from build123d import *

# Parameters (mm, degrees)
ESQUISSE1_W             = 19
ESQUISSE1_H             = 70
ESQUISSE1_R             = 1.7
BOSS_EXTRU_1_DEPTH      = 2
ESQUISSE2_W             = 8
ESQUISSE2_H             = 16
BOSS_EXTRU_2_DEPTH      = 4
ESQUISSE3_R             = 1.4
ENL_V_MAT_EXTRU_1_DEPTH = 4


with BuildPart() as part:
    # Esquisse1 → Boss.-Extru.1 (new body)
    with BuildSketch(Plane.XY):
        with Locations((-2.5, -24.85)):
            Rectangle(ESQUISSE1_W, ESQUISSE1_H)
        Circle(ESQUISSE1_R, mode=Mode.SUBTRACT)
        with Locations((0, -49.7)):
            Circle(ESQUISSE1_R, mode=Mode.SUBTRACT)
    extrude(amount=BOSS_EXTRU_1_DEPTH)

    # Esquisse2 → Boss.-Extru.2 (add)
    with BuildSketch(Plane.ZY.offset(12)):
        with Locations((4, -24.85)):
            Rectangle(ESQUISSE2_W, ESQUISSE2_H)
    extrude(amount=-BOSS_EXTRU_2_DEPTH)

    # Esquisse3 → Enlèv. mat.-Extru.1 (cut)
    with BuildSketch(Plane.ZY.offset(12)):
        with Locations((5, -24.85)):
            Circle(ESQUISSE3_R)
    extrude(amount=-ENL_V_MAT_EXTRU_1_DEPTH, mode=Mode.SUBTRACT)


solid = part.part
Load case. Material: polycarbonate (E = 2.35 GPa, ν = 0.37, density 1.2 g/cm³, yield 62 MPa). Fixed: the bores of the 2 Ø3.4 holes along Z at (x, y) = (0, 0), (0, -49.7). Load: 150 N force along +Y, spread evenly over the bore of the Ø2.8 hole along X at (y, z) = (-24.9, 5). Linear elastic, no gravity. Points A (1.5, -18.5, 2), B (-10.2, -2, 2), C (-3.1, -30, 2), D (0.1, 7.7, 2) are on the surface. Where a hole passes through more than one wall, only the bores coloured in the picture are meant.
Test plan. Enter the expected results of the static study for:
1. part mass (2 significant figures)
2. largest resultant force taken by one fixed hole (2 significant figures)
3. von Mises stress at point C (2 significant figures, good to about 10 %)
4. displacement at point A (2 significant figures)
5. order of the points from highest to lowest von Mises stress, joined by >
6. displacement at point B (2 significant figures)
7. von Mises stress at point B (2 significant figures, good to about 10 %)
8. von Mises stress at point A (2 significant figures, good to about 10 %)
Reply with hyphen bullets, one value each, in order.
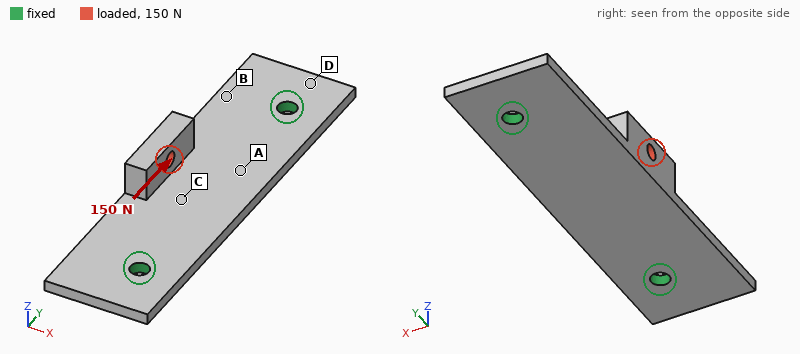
- 3.6 g
- 82 N
- 10 MPa
- 0.090 mm
- C > A > B > D
- 0.12 mm
- 3.6 MPa
- 6.9 MPa
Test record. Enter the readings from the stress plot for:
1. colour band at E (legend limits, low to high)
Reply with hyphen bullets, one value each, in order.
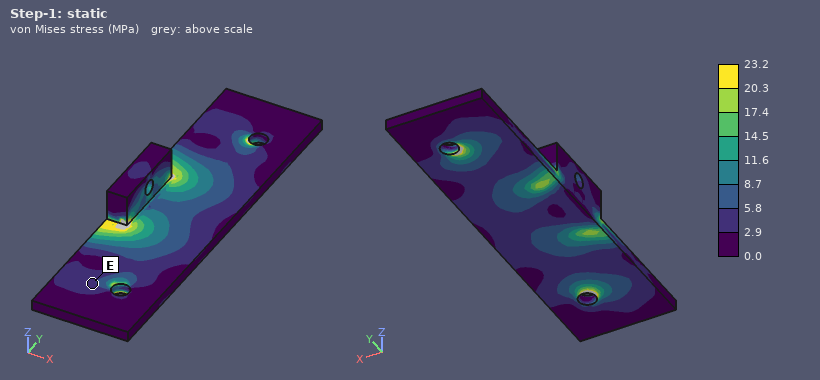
- 2.9 to 5.8 MPa
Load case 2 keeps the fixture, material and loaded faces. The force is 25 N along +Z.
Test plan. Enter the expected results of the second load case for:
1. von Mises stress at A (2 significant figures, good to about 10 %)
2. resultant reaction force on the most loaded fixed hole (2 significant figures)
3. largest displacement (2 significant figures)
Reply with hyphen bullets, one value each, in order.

- 3.4 MPa
- 13 N
- 0.74 mm
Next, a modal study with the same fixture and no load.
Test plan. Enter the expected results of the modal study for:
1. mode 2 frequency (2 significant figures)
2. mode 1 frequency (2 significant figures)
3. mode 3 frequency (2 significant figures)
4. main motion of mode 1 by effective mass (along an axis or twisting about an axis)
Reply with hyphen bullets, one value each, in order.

- 1600 Hz
- 1000 Hz
- 2600 Hz
- along Z
